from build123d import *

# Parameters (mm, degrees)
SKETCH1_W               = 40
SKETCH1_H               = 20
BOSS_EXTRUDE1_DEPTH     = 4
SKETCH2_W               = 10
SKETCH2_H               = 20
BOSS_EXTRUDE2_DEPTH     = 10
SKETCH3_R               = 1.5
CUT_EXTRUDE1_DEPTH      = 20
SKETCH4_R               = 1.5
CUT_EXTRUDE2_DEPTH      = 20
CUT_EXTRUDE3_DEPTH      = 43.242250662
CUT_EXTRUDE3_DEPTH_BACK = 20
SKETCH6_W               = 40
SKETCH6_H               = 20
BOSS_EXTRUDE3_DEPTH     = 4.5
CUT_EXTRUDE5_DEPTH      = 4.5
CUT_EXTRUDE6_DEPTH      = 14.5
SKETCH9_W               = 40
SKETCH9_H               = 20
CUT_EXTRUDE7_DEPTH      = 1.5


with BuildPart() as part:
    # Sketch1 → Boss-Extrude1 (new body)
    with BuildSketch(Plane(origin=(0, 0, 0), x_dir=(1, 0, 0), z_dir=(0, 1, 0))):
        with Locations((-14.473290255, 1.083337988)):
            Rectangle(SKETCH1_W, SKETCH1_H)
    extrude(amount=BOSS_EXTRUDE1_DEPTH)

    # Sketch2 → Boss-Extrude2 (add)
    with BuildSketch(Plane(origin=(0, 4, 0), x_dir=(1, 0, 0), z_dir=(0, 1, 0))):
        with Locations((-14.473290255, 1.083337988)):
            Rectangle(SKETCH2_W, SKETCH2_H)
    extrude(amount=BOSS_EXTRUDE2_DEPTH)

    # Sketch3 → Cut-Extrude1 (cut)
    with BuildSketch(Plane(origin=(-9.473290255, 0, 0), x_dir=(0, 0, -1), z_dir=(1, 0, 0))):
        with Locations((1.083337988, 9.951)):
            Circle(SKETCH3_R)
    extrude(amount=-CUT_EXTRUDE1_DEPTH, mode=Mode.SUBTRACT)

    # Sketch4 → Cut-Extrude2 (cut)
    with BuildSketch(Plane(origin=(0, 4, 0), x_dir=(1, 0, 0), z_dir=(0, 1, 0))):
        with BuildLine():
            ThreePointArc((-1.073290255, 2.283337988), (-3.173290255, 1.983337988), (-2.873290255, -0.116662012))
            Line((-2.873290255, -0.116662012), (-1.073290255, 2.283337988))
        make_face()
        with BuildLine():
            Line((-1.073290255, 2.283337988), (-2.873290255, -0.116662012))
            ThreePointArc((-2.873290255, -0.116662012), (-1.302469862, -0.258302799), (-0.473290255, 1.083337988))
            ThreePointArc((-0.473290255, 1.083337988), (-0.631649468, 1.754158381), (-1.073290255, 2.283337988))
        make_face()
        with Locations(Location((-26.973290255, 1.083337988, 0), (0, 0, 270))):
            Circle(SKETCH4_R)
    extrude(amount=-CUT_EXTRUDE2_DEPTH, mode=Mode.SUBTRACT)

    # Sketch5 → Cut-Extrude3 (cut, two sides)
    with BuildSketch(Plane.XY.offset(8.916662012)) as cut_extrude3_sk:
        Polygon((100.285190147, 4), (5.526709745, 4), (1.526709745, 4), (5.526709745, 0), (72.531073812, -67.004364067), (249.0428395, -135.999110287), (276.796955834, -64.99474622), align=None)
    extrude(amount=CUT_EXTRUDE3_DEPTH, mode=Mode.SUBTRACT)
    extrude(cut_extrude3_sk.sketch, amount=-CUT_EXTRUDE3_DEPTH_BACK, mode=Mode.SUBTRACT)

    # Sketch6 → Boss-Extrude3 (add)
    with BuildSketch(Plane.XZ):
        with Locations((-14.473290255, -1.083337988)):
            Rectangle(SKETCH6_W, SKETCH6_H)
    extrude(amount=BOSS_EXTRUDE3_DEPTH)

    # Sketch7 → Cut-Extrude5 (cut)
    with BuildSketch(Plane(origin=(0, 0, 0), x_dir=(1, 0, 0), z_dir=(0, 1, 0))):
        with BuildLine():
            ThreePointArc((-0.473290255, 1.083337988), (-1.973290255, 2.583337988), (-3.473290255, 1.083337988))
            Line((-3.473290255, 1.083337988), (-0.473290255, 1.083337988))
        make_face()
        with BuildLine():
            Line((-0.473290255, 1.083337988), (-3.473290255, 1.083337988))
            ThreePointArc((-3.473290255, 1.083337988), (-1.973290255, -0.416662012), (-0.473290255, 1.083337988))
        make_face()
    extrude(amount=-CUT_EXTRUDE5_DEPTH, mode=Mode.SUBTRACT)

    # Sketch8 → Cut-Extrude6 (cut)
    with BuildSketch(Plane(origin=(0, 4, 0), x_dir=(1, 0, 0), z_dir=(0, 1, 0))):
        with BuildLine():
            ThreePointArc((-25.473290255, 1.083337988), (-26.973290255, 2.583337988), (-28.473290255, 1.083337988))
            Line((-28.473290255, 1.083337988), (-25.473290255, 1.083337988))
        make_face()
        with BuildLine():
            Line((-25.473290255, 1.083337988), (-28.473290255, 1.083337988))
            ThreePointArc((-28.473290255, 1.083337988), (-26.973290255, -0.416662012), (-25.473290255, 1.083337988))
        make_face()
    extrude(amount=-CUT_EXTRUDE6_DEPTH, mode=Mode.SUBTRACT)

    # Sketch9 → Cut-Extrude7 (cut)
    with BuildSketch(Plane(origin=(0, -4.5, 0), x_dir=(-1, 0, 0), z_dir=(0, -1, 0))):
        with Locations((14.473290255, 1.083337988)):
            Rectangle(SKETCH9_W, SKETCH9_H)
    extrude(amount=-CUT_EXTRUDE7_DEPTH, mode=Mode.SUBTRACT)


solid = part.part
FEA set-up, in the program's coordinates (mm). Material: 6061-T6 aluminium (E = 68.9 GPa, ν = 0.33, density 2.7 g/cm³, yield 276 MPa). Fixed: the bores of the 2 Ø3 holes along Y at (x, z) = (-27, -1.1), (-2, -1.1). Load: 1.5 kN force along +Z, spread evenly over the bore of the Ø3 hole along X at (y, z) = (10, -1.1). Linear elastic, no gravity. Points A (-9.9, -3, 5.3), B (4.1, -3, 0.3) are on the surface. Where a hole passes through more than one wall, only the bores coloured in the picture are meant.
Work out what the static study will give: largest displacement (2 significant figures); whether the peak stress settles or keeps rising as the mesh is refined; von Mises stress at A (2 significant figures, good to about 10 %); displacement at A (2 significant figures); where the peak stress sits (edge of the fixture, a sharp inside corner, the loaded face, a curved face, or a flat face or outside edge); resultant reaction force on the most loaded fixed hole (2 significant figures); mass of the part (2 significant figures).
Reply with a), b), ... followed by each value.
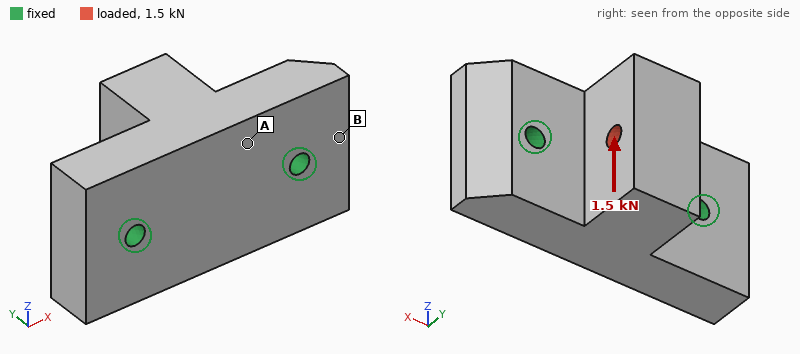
a) 31 µm
b) keeps rising
c) 21 MPa
d) 8.9 µm
e) edge of the fixture
f) 750 N
g) 20 g
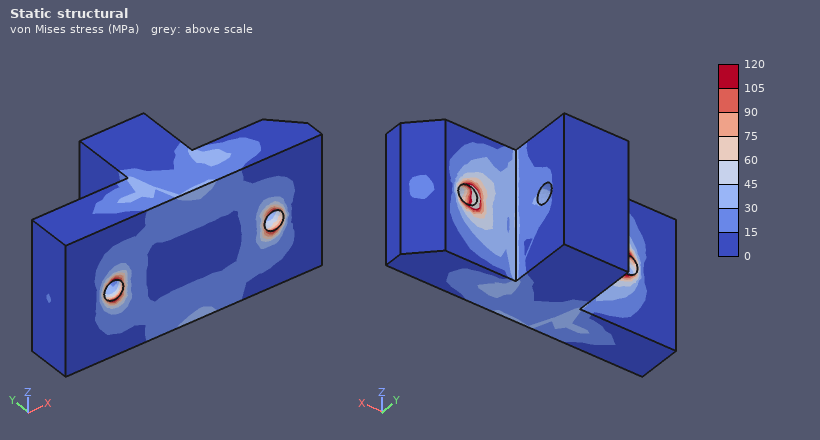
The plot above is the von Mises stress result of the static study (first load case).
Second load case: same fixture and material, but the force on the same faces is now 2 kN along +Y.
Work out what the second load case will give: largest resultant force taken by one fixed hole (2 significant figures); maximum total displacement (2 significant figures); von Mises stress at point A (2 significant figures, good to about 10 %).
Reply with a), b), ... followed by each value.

a) 1.0 kN
b) 10 µm
c) 16 MPa
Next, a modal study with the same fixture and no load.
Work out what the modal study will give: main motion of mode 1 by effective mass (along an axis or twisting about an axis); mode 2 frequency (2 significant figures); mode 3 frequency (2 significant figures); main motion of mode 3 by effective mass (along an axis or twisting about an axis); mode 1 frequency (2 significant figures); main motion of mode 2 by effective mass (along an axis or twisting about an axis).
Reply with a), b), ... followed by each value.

a) along Z
b) 25 kHz
c) 28 kHz
d) along X
e) 16 kHz
f) along Y
